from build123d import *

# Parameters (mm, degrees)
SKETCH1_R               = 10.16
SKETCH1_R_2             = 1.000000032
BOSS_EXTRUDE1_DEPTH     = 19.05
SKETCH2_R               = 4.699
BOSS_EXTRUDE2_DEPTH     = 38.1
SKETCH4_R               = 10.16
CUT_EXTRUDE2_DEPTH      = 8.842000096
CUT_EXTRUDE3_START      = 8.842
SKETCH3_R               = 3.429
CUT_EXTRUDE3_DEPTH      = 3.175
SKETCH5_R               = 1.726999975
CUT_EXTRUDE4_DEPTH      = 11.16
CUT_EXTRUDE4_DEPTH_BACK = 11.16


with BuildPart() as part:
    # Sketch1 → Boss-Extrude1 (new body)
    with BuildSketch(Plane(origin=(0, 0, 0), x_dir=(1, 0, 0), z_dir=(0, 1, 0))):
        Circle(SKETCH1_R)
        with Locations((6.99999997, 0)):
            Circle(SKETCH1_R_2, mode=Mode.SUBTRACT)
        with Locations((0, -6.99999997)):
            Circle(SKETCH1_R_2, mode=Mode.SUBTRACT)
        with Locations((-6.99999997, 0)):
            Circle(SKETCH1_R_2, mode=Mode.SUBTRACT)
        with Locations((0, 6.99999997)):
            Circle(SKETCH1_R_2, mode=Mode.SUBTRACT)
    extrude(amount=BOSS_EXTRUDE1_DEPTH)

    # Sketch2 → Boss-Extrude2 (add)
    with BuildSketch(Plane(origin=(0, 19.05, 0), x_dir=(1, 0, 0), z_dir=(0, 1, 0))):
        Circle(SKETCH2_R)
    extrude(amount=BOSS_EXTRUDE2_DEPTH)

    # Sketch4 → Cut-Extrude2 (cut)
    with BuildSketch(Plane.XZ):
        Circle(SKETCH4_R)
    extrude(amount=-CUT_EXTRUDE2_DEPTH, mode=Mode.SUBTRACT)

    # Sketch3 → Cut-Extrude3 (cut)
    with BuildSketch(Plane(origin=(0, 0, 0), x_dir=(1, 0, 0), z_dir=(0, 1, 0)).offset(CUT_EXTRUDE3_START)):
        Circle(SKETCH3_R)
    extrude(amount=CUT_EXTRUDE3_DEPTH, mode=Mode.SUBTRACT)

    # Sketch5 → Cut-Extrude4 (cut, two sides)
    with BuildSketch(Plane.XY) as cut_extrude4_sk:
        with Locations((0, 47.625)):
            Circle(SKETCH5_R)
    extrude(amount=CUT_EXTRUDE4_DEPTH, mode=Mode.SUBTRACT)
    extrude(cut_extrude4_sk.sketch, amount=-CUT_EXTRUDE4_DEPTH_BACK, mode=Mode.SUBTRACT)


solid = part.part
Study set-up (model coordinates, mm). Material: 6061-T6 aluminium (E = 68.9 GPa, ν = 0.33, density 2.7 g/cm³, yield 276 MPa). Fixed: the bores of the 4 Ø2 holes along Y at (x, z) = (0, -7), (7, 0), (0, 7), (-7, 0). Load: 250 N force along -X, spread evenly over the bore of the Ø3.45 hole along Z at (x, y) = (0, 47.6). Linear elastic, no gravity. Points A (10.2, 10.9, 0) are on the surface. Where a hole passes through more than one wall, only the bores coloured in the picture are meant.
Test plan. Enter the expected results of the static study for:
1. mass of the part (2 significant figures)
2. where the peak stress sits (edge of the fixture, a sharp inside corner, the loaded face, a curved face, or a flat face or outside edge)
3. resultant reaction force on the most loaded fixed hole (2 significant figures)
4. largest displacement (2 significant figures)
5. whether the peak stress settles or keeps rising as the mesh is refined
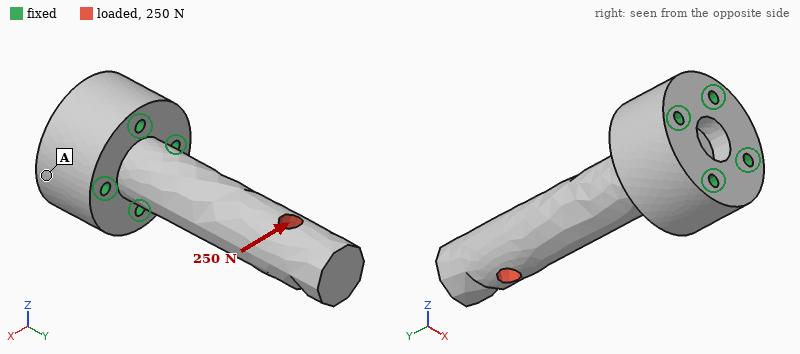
15 g
a sharp inside corner
530 N
0.14 mm
keeps rising
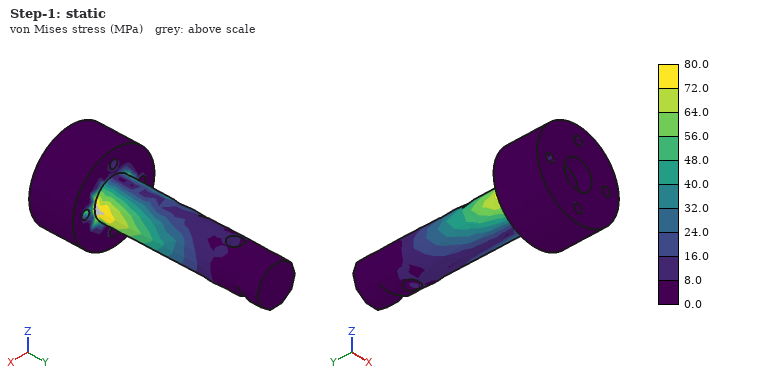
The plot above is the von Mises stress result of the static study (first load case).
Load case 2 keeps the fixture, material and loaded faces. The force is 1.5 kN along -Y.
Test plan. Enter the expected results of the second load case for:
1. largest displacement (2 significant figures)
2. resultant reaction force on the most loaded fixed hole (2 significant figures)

12 µm
410 N
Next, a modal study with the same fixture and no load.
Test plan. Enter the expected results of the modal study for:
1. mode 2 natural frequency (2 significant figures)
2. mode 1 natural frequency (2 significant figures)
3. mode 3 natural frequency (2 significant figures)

4200 Hz
4100 Hz
20 kHz
